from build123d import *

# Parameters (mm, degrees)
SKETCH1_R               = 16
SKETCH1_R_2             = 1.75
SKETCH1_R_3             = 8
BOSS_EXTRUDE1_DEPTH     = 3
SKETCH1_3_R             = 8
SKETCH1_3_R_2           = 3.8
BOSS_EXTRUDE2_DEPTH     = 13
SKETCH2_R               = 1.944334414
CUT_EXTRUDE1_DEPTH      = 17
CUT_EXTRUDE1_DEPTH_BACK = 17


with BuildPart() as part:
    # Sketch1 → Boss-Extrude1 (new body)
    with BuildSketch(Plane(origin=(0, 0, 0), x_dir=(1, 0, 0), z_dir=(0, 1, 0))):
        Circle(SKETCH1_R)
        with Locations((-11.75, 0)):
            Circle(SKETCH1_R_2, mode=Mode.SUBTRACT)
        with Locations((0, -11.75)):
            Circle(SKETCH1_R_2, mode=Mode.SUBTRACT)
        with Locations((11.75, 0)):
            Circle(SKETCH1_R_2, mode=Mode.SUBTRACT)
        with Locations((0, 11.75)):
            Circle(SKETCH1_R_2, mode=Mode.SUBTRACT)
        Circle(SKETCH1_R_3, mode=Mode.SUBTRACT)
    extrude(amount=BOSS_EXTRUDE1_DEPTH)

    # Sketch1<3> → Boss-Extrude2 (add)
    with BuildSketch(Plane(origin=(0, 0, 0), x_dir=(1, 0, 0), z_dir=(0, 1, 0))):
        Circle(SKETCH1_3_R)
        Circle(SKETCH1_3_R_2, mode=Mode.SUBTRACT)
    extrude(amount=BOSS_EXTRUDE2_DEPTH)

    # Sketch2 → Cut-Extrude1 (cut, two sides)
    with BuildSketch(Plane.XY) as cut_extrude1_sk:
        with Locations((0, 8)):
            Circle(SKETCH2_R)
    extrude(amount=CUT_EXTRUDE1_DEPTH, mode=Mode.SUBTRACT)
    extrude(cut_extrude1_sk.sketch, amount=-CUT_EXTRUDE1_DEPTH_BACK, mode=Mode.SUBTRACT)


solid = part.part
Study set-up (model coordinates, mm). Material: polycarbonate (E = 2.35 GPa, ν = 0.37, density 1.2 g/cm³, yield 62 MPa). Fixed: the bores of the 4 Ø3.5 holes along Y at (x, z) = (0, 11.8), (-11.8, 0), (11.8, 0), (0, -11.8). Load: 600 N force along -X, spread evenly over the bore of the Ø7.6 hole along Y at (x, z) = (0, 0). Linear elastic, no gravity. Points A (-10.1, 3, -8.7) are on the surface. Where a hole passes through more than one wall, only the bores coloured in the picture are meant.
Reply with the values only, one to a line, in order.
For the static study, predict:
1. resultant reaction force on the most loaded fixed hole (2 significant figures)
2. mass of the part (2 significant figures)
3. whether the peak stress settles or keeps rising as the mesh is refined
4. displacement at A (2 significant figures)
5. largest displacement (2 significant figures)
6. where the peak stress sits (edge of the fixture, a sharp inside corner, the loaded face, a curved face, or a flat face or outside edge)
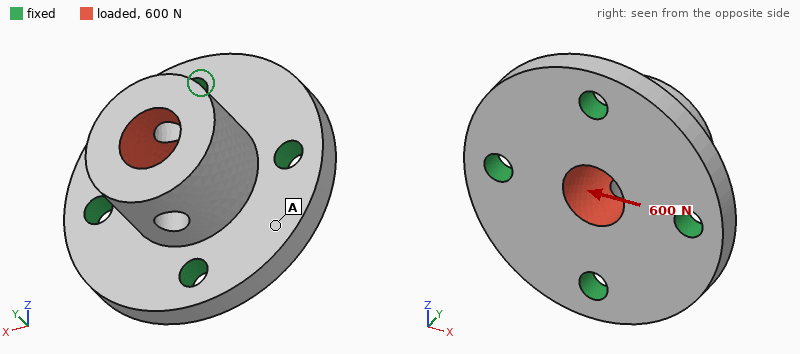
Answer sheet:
240 N
4.3 g
keeps rising
0.019 mm
0.12 mm
edge of the fixture
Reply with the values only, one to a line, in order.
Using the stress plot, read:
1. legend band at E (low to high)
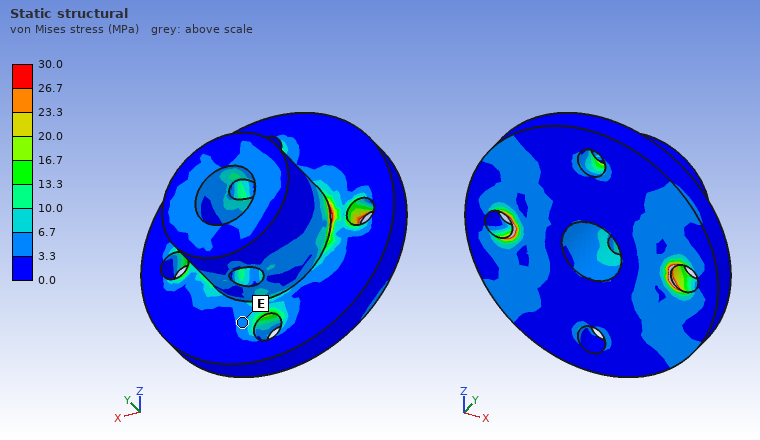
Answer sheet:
3.3 to 6.7 MPa
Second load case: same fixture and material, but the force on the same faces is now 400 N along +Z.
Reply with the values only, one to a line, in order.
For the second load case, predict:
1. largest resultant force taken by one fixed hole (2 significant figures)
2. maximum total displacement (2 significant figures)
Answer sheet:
160 N
76 µm
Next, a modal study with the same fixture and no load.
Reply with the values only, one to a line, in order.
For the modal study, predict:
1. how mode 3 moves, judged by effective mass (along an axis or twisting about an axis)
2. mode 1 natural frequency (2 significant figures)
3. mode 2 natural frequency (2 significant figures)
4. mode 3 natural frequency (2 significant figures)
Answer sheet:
along Y
8400 Hz
8500 Hz
10 kHz
